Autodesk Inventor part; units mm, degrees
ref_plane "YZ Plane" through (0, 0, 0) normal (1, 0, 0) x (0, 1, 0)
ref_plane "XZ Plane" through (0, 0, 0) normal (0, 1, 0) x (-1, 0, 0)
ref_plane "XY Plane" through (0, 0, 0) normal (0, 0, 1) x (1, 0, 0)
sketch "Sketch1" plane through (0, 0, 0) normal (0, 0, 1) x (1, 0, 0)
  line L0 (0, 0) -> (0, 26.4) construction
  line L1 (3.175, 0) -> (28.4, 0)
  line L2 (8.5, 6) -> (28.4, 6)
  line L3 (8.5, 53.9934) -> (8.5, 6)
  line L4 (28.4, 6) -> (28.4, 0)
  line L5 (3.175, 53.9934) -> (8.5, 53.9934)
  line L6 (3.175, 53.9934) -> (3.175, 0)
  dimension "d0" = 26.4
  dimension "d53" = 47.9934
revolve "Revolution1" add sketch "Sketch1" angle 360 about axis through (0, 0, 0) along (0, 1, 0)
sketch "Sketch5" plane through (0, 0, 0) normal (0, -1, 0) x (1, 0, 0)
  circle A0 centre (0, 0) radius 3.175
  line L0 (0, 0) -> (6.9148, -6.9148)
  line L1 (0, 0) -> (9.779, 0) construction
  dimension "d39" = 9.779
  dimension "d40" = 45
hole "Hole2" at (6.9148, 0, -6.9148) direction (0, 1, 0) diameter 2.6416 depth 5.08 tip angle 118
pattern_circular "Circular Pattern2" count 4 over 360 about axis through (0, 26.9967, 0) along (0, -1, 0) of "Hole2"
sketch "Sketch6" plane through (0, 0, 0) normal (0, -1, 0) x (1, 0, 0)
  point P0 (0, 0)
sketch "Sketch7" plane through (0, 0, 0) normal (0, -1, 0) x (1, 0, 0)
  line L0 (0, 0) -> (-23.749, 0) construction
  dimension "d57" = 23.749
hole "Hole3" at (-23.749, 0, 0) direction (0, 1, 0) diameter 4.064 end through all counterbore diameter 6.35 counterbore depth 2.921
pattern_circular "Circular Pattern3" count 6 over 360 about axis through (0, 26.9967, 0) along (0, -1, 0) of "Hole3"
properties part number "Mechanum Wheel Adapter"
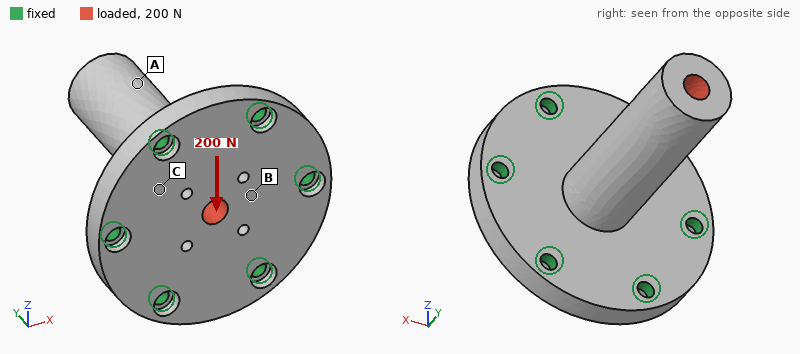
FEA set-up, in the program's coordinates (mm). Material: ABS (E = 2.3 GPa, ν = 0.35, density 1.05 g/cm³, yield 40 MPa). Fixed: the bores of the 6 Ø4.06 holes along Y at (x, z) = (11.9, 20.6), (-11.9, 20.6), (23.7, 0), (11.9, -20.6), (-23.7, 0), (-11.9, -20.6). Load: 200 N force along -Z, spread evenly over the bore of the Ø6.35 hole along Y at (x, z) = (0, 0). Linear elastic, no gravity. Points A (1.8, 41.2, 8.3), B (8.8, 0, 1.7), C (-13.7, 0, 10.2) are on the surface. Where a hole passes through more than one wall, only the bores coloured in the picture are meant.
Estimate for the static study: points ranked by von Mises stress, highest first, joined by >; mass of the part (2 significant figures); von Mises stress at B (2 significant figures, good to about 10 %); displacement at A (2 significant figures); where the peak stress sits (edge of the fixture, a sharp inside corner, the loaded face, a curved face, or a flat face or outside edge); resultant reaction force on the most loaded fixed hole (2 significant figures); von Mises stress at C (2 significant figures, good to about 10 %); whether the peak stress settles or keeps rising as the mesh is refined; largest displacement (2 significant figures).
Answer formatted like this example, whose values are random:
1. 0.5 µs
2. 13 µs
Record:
1. B > C > A
2. 25 g
3. 4.4 MPa
4. 0.51 mm
5. edge of the fixture
6. 71 N
7. 2.5 MPa
8. keeps rising
9. 0.70 mm
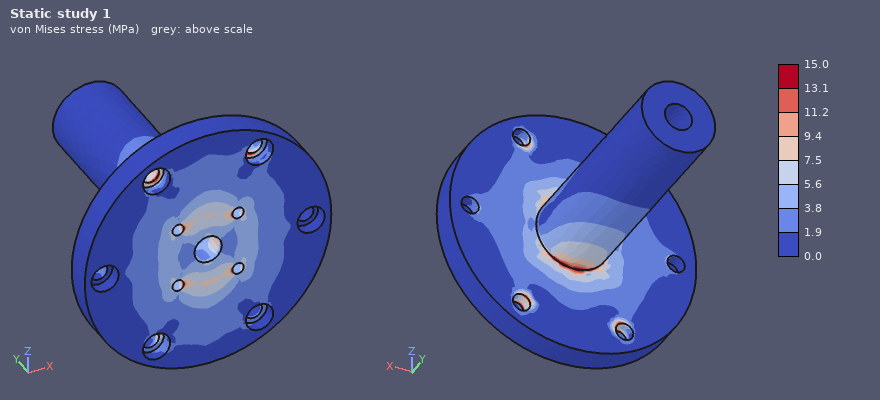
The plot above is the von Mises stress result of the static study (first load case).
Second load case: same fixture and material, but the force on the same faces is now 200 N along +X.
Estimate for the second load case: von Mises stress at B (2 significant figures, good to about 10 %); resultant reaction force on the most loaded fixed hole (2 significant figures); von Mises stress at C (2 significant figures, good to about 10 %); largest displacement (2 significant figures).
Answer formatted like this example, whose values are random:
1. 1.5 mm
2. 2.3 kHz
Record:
1. 7.5 MPa
2. 79 N
3. 2.7 MPa
4. 0.70 mm
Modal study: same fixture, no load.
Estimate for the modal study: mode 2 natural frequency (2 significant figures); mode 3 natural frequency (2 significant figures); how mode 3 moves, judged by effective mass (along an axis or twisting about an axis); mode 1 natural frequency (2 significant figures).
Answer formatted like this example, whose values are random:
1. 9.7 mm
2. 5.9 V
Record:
1. 990 Hz
2. 2700 Hz
3. along Y
4. 990 Hz
